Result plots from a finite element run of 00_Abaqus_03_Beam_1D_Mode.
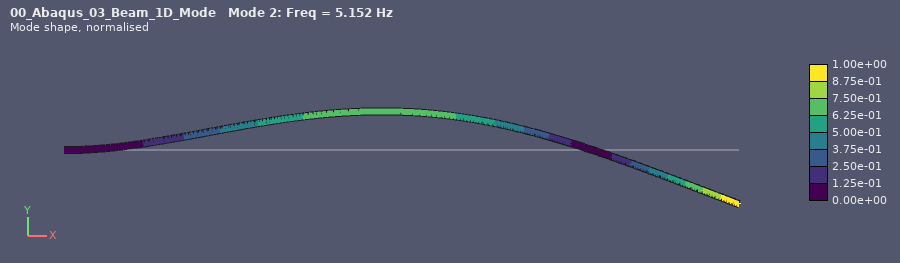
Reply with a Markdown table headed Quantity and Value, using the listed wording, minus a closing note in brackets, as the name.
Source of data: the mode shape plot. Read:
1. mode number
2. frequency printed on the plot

| Quantity | Value |
|---|---|
| mode number | 2 |
| frequency printed on the plot | 5.152 Hz |
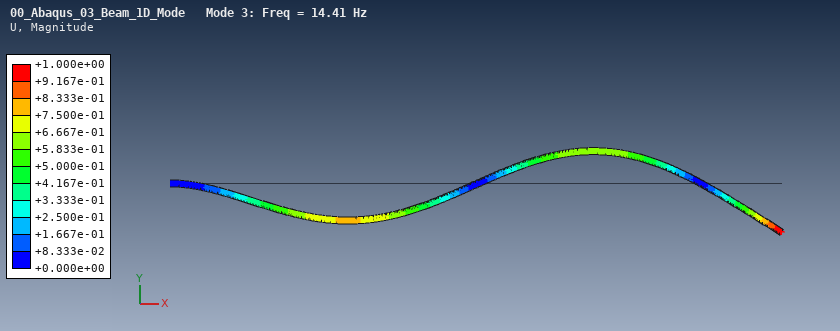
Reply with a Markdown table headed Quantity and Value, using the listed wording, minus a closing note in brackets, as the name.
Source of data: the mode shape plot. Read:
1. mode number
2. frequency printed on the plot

| Quantity | Value |
|---|---|
| mode number | 3 |
| frequency printed on the plot | 14.41 Hz |
